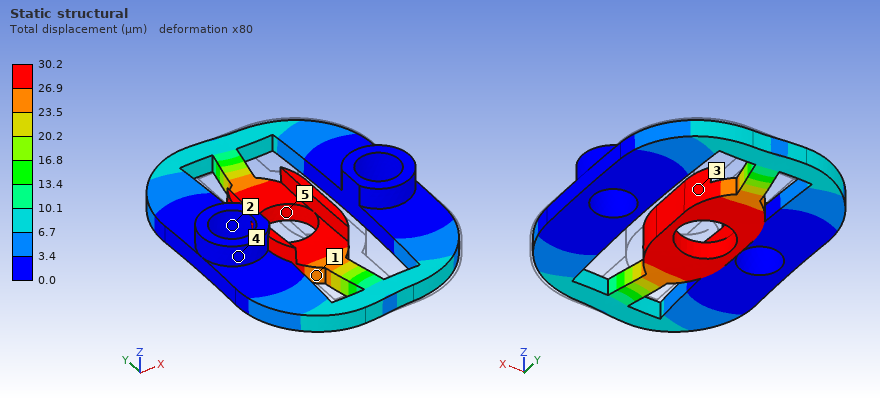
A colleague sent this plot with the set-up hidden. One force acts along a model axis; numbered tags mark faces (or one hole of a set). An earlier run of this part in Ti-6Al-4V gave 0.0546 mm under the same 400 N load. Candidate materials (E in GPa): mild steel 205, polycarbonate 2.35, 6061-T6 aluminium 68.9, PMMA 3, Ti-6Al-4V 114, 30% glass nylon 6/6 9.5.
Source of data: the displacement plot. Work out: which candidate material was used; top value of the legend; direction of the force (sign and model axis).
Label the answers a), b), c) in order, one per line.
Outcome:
a) mild steel
b) 30.2 µm
c) -X
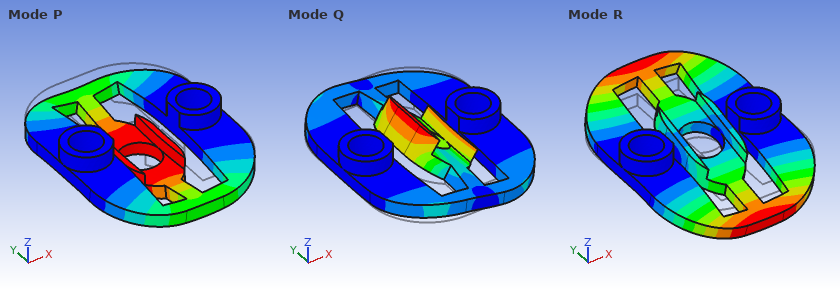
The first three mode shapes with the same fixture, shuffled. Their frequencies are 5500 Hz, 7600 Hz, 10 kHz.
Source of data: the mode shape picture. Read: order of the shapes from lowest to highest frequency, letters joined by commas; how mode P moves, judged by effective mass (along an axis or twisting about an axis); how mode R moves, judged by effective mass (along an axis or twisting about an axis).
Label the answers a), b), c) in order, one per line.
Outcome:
a) P, R, Q
b) along Z
c) twisting about X
